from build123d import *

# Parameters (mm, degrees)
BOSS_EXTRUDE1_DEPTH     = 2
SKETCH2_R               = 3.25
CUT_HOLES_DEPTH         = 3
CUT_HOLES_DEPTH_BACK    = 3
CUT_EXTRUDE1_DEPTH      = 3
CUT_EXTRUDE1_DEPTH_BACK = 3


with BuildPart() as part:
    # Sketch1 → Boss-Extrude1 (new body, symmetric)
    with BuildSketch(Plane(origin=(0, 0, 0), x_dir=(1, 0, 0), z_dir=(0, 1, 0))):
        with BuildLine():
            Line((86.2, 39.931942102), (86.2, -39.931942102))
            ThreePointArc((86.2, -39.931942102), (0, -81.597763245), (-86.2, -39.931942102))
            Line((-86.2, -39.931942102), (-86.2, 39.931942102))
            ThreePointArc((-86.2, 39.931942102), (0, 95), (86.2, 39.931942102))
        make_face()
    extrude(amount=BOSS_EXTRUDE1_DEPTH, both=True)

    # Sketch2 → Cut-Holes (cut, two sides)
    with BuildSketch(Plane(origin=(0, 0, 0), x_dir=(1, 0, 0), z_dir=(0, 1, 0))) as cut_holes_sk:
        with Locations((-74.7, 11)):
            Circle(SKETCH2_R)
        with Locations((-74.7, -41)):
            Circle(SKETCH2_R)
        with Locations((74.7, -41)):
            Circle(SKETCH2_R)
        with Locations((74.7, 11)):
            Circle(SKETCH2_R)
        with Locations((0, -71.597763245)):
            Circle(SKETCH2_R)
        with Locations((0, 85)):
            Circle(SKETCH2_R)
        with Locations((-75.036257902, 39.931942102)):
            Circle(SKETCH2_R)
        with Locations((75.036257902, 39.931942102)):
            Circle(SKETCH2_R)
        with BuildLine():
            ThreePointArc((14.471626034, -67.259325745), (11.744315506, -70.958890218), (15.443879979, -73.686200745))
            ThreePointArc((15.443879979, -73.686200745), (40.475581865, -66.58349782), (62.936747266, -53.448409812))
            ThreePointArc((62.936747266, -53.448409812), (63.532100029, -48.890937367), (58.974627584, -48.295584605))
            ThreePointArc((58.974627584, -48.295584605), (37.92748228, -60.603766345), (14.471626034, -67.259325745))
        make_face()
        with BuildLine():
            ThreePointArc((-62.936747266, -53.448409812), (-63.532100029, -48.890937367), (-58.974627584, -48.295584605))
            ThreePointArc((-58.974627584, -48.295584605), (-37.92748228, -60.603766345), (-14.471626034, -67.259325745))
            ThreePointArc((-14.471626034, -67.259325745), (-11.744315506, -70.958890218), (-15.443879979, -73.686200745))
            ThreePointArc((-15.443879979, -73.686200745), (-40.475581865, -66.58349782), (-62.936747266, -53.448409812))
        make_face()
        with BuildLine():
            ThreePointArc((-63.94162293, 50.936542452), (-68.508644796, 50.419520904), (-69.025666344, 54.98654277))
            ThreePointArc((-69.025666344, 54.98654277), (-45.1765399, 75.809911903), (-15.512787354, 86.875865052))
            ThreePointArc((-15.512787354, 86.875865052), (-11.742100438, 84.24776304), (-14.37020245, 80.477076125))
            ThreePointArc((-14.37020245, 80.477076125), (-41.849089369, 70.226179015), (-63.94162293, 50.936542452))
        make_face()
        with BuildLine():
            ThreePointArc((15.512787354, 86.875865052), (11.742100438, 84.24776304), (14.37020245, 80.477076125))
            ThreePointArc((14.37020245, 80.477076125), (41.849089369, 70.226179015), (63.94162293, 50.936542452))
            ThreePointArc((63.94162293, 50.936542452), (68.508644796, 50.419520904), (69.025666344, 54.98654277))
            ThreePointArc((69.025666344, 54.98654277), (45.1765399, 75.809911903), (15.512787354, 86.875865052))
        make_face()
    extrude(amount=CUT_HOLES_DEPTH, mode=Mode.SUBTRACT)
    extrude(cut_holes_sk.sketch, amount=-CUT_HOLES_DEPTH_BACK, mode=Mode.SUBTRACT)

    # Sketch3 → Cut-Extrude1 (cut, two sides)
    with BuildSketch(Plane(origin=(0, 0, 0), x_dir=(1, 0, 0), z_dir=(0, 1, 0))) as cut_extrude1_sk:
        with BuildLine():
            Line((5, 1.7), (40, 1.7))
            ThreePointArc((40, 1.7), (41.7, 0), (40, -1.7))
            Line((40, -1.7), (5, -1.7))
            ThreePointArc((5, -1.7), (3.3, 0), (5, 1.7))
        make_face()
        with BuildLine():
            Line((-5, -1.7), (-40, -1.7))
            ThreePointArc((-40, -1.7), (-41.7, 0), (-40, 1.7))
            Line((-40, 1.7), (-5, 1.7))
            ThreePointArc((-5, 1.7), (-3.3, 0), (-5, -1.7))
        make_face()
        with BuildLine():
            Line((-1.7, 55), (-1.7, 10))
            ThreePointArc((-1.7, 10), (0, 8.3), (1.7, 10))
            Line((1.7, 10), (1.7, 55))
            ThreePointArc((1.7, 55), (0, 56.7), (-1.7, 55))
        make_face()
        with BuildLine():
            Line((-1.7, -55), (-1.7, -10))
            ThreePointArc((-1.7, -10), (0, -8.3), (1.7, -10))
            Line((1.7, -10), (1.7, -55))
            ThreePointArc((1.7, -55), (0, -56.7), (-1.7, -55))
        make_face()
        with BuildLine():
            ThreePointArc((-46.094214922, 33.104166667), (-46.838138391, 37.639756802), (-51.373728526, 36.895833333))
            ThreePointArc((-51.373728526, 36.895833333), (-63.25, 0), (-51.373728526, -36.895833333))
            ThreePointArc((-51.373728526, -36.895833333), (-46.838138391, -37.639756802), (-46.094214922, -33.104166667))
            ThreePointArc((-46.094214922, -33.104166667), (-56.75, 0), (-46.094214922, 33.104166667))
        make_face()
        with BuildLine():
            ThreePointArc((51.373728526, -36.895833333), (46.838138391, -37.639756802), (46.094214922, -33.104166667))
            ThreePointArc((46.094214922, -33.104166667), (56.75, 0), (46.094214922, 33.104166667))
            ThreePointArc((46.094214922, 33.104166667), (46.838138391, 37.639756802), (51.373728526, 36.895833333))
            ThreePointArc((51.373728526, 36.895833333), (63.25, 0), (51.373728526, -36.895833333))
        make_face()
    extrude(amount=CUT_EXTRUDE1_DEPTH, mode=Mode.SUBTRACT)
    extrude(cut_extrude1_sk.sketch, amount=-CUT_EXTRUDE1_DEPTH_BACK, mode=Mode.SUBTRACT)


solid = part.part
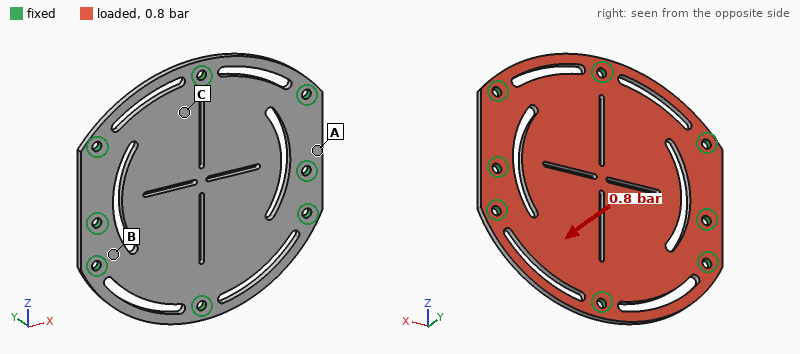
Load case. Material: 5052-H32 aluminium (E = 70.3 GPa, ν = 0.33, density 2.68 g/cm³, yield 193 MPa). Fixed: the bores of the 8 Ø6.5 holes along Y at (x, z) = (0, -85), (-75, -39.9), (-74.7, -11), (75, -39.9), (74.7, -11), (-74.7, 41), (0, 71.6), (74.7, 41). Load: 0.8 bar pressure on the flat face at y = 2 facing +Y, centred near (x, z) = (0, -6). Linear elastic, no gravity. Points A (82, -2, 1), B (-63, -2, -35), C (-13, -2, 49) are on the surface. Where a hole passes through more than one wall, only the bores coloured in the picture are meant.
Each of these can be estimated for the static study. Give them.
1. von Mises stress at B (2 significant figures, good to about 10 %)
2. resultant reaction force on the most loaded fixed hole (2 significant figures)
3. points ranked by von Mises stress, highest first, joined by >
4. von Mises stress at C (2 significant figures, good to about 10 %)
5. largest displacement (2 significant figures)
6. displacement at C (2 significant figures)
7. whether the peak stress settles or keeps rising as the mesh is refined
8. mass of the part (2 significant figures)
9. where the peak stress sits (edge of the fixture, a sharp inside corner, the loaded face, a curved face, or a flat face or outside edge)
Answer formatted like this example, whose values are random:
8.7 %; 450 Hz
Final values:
29 MPa; 350 N; B > C > A; 15 MPa; 0.34 mm; 0.085 mm; keeps rising; 240 g; edge of the fixture
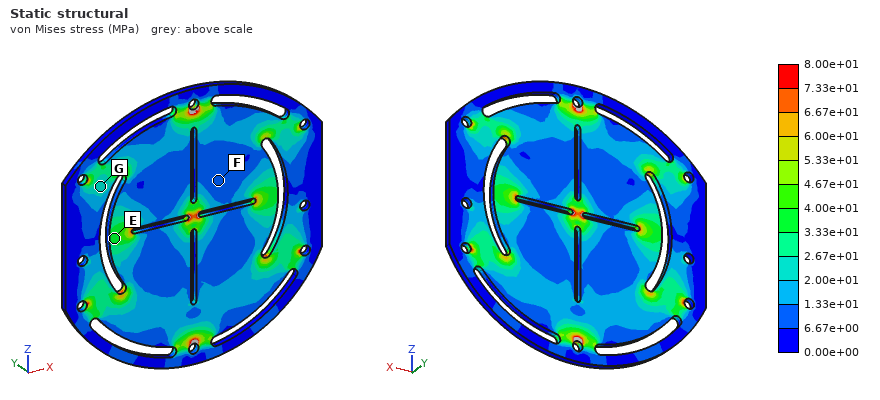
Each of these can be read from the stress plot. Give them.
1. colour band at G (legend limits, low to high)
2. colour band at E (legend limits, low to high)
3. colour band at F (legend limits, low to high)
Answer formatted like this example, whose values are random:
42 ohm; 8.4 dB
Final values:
2.00e+01 to 2.67e+01 MPa; 3.33e+01 to 4.00e+01 MPa; 6.67e+00 to 1.33e+01 MPa
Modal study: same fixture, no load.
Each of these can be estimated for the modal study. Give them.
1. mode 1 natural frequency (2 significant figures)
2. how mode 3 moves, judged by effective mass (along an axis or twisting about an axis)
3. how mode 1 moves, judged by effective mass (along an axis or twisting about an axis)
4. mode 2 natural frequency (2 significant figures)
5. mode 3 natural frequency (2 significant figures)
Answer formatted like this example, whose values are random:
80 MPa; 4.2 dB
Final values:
930 Hz; twisting about X; along Y; 1600 Hz; 2300 Hz
